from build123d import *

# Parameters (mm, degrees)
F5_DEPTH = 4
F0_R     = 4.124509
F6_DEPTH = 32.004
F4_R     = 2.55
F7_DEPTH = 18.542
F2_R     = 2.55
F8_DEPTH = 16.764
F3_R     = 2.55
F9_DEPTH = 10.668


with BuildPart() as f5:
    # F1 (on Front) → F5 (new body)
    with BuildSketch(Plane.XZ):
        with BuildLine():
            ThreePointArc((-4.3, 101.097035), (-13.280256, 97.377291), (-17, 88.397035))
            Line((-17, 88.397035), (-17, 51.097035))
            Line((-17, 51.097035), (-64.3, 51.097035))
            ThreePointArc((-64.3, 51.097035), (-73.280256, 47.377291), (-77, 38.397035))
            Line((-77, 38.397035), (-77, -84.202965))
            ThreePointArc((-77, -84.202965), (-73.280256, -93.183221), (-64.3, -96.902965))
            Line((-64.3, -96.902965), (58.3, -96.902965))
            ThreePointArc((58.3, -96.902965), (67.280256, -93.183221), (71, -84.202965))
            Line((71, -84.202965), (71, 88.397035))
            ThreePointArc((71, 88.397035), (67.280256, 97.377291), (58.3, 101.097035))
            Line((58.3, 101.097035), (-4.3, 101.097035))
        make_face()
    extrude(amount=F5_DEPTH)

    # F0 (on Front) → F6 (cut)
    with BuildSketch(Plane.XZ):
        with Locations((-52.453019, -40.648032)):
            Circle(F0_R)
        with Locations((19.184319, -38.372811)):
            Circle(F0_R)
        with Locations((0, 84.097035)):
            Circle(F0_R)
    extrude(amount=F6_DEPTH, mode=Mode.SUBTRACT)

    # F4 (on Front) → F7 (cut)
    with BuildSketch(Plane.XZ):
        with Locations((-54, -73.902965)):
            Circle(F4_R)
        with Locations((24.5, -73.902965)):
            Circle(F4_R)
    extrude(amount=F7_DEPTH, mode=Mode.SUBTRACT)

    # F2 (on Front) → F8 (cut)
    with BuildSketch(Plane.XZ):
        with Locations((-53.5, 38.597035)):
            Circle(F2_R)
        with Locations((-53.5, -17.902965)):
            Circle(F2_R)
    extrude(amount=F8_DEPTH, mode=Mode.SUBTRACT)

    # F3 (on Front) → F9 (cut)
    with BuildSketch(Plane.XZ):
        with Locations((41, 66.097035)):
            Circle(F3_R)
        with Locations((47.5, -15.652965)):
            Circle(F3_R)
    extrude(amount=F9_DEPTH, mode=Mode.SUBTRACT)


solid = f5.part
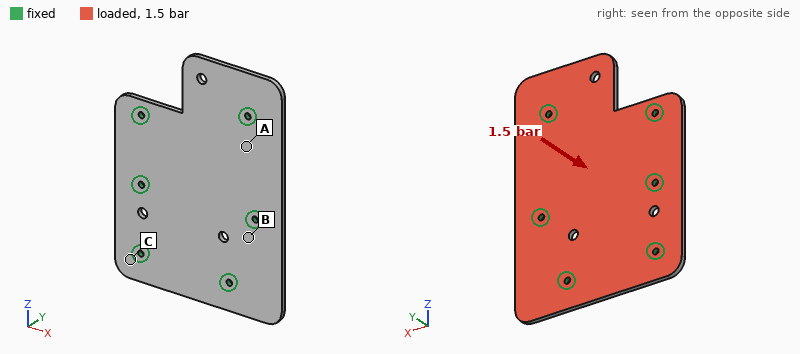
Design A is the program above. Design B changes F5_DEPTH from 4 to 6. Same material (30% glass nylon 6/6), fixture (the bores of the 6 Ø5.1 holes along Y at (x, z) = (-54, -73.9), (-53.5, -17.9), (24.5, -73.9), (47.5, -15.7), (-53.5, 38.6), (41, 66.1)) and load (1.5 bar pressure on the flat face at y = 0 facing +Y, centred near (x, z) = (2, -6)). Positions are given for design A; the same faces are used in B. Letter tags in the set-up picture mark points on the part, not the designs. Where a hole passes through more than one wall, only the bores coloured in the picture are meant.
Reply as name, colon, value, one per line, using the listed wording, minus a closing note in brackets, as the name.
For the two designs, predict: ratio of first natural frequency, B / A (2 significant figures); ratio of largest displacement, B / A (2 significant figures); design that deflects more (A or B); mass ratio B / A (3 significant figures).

ratio of first natural frequency, B / A: 1.4
ratio of largest displacement, B / A: 0.32
design that deflects more: A
mass ratio B / A: 1.50
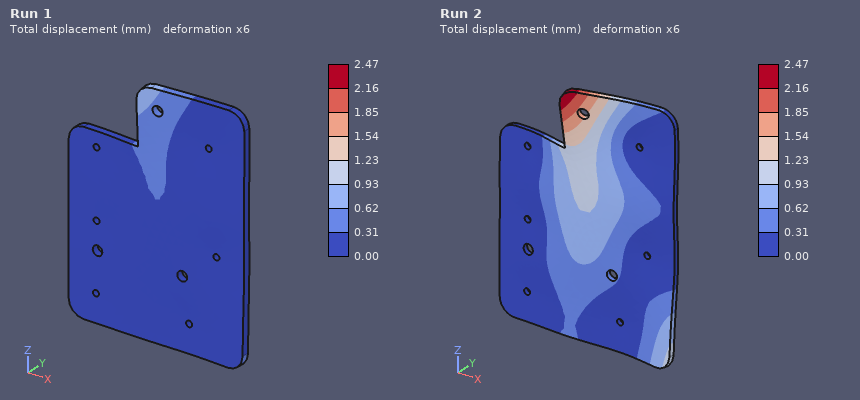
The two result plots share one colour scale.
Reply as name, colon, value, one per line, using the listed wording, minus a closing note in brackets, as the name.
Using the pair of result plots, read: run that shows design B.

run that shows design B: Run 1
